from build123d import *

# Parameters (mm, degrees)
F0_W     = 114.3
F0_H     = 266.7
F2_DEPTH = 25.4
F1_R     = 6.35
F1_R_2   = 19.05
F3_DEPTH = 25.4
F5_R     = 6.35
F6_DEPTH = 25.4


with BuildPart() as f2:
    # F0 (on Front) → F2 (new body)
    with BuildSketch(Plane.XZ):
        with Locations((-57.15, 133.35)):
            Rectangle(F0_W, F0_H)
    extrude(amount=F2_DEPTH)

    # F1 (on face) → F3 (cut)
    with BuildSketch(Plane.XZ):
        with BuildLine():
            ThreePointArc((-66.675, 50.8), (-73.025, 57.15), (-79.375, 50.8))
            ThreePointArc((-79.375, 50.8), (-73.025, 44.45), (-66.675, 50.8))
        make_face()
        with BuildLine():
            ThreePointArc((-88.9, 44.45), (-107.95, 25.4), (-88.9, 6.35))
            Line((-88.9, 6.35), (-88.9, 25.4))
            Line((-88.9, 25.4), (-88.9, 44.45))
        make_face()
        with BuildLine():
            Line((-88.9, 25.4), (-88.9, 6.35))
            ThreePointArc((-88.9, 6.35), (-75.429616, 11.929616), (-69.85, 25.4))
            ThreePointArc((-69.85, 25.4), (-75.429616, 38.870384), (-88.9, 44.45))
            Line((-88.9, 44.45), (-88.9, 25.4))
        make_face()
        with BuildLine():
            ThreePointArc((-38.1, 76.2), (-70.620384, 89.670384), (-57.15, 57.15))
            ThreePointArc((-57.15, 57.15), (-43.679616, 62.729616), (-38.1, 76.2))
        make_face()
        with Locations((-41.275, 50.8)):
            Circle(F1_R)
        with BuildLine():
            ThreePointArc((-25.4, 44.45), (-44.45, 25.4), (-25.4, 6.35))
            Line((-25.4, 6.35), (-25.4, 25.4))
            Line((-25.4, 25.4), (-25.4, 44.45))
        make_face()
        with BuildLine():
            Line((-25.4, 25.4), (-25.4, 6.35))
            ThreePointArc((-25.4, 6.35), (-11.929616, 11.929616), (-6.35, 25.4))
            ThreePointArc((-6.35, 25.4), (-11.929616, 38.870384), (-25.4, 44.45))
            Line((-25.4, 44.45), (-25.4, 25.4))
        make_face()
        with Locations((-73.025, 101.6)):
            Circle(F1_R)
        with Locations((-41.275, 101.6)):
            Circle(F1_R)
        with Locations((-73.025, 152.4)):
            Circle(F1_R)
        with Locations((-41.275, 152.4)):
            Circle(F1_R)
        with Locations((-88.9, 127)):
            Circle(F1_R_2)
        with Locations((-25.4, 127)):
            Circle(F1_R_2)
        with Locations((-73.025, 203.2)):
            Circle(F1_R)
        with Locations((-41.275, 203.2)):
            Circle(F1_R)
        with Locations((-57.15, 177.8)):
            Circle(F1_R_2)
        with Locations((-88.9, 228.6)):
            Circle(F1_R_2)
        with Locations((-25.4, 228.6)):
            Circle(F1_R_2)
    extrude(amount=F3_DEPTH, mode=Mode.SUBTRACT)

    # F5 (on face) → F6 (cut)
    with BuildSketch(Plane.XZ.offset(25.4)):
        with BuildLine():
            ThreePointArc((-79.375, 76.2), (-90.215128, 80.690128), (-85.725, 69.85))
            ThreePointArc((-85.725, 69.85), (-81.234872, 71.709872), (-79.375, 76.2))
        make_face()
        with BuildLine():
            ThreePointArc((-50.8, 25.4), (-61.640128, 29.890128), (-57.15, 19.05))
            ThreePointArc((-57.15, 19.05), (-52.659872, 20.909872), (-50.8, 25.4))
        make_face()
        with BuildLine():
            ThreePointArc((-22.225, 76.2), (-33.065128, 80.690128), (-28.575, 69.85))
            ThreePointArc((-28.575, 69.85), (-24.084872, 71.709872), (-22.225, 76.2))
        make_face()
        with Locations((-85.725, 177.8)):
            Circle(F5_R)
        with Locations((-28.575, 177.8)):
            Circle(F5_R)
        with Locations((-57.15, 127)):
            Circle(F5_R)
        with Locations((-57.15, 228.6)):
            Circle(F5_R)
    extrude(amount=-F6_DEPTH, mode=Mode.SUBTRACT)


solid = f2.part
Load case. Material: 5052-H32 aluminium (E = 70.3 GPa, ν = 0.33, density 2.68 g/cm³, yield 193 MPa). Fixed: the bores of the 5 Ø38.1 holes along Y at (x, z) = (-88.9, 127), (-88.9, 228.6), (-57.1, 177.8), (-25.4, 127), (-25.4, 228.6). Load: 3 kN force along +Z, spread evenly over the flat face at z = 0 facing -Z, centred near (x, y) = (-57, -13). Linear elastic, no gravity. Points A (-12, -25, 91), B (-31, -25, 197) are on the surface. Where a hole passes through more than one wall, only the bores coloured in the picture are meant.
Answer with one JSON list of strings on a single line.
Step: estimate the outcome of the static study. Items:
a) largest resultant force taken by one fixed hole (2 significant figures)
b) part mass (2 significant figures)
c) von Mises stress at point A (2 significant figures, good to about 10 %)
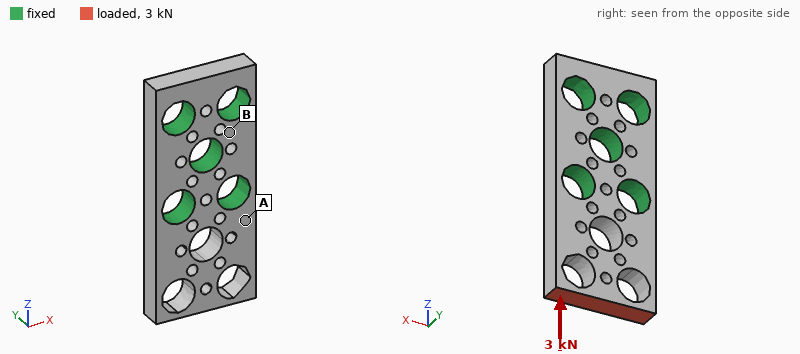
["1.5 kN", "1.3 kg", "2.0 MPa"]
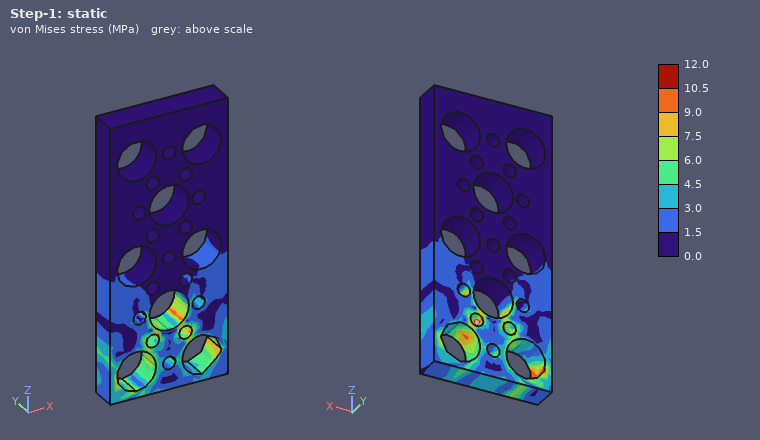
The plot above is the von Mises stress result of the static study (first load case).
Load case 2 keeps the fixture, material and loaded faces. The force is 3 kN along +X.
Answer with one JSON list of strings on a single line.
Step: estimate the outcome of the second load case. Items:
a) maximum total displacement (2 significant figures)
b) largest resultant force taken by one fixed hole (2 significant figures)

["38 µm", "3.8 kN"]
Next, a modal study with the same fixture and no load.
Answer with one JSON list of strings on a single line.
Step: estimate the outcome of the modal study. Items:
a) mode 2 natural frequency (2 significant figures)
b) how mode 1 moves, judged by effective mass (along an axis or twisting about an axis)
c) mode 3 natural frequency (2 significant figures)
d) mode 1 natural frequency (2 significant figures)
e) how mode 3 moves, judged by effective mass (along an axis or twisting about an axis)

["3100 Hz", "along Y", "3700 Hz", "1600 Hz", "along X"]
